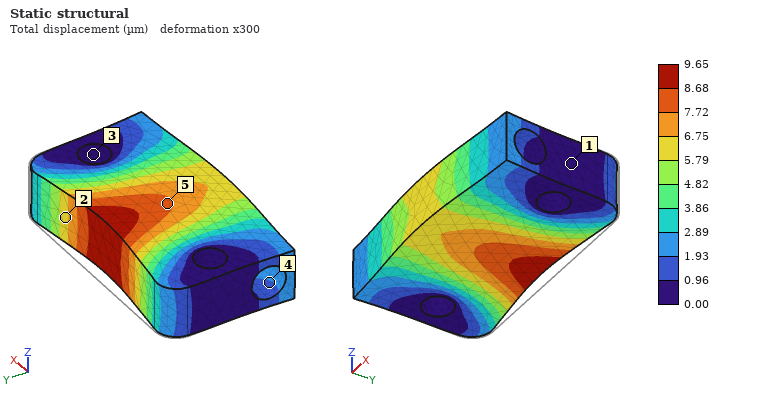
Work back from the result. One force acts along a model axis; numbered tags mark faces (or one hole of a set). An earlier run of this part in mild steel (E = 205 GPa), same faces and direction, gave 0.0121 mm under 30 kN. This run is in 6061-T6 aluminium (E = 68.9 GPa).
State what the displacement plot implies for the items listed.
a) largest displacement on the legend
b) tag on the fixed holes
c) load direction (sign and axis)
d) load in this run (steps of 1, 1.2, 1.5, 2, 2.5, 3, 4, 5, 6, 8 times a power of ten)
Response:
9.65 µm
3
-Y
8 kN
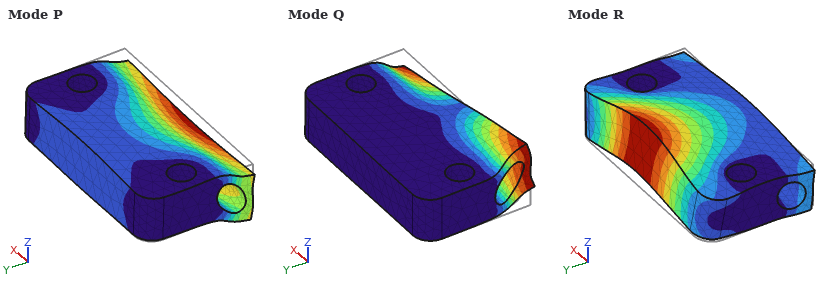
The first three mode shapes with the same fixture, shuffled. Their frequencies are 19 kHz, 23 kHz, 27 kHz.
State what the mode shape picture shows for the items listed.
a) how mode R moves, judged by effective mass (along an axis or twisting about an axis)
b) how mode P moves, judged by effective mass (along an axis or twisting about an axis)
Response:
along Z
along Z
